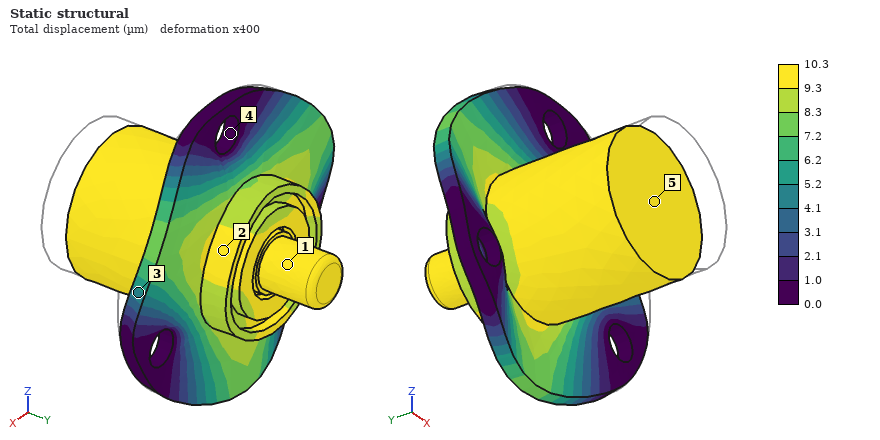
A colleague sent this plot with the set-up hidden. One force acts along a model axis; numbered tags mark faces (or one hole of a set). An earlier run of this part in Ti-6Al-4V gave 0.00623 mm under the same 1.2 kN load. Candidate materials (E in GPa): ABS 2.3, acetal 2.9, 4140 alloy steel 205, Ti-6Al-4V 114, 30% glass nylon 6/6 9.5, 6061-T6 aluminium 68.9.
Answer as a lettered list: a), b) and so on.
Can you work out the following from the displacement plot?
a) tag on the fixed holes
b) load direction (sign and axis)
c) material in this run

a) 4
b) +Y
c) 6061-T6 aluminium
